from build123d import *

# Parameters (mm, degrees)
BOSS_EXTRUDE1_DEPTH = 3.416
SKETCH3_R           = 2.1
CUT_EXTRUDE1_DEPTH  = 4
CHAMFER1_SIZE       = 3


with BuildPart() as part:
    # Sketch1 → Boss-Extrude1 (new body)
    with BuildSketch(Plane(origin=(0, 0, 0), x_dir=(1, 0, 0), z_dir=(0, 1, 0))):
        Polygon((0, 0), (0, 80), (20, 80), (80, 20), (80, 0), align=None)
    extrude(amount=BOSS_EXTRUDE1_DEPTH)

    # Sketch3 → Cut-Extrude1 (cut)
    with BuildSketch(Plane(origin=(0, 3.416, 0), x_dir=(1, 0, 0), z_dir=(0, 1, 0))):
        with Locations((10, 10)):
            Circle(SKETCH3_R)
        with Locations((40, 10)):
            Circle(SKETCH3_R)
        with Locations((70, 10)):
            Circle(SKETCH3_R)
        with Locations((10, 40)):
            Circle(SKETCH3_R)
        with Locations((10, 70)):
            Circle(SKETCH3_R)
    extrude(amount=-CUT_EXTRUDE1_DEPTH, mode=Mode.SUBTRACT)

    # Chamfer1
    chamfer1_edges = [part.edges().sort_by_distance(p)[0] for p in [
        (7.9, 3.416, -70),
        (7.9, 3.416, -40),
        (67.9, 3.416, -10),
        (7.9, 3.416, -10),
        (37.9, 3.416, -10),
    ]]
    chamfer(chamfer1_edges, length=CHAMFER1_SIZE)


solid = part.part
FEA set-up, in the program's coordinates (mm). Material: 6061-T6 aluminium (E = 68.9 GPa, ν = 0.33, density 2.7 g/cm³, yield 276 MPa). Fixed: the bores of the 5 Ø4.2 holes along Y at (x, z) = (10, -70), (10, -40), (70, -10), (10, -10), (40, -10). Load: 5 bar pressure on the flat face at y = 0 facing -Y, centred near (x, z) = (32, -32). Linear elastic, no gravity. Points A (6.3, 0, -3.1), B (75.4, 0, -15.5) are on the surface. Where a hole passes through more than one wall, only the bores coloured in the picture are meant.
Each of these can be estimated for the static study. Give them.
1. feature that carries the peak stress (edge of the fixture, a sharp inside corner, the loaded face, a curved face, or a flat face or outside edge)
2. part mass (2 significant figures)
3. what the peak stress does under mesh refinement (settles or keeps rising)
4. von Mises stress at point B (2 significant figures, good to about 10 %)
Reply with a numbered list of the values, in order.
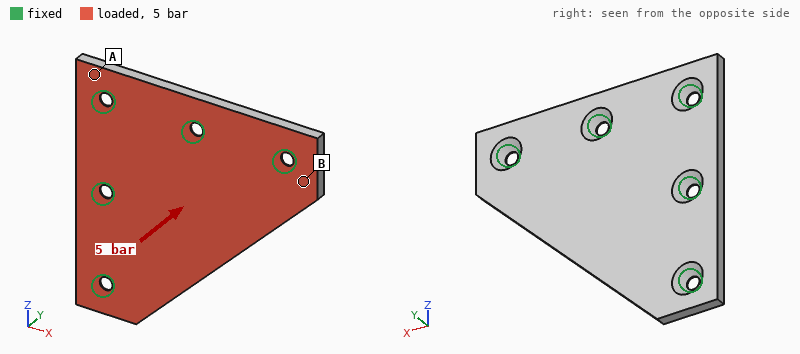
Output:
1. edge of the fixture
2. 41 g
3. keeps rising
4. 60 MPa
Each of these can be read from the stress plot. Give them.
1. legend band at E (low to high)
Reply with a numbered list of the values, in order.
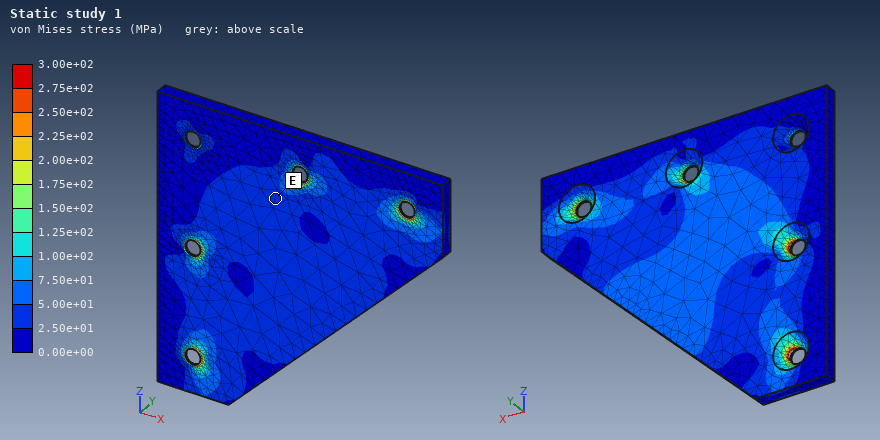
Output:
1. 2.50e+01 to 5.00e+01 MPa
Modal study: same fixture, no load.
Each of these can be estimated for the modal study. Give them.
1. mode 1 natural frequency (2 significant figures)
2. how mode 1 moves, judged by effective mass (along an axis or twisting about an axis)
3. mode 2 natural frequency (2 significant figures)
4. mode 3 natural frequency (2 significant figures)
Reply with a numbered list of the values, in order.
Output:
1. 2400 Hz
2. along Y
3. 5100 Hz
4. 8400 Hz
